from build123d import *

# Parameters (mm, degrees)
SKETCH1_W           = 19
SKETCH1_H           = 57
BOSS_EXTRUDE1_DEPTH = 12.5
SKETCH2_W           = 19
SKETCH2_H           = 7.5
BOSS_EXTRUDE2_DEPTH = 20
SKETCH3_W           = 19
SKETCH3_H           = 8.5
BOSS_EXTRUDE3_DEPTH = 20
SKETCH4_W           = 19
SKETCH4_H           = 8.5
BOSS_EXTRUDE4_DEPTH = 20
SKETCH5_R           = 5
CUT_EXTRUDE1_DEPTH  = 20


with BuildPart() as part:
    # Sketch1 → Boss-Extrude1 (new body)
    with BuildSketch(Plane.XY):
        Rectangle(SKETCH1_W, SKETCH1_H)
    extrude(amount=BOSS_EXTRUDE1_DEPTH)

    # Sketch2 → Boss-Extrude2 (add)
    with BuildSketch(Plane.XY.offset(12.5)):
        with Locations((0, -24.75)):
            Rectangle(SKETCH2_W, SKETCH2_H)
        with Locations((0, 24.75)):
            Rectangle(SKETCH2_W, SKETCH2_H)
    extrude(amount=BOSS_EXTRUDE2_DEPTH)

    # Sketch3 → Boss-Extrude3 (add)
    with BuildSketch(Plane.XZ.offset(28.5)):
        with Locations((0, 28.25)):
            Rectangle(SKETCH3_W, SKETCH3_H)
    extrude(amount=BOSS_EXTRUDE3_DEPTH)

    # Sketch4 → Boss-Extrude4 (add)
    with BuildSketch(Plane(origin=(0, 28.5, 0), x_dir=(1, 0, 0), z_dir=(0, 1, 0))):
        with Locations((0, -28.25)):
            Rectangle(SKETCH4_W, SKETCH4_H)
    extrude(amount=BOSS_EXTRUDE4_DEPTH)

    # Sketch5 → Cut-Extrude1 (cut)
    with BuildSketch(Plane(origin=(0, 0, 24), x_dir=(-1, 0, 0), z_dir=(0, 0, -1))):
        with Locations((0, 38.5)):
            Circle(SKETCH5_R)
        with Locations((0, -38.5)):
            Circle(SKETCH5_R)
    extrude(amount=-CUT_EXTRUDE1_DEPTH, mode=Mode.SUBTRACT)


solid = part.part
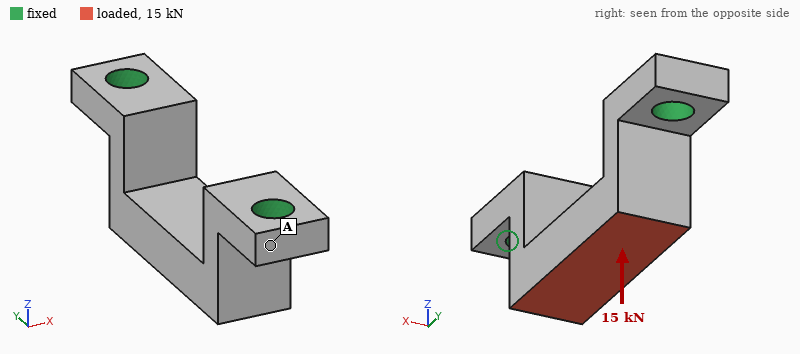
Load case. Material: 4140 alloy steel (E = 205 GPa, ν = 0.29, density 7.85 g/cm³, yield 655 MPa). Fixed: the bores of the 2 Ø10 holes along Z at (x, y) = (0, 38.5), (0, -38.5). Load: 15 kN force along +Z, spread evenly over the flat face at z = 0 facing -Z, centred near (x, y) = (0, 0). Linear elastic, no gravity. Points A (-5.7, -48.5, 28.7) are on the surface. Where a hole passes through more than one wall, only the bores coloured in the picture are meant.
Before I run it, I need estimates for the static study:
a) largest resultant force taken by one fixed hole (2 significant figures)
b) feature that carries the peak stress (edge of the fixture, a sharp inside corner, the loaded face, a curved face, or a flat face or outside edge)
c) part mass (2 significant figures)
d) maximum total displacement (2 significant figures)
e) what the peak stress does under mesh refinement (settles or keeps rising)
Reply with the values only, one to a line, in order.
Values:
8.3 kN
edge of the fixture
190 g
30 µm
keeps rising
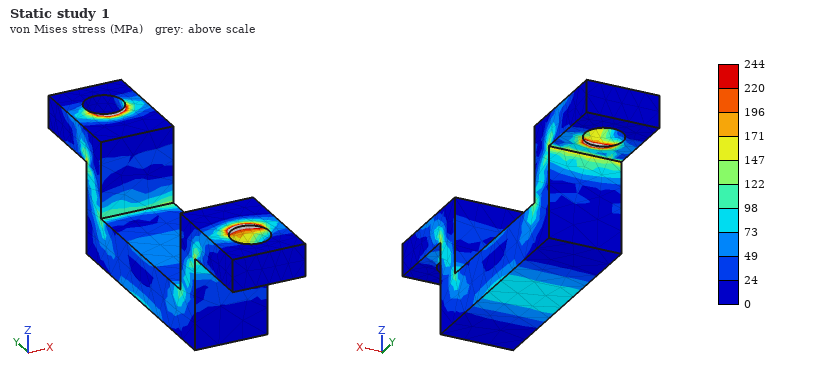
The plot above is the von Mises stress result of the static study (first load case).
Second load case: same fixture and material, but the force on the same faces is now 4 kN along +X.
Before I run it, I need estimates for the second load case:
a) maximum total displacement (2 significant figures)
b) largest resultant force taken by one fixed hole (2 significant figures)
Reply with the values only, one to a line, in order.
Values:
77 µm
2.0 kN
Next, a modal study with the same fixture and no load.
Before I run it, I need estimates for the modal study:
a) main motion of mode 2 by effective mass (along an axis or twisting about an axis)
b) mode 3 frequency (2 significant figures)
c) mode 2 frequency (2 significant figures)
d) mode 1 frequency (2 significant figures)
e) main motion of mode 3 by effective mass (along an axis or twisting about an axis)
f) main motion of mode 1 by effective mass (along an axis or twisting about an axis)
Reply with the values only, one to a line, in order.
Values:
along Y
9100 Hz
7300 Hz
4400 Hz
twisting about Z
along X
